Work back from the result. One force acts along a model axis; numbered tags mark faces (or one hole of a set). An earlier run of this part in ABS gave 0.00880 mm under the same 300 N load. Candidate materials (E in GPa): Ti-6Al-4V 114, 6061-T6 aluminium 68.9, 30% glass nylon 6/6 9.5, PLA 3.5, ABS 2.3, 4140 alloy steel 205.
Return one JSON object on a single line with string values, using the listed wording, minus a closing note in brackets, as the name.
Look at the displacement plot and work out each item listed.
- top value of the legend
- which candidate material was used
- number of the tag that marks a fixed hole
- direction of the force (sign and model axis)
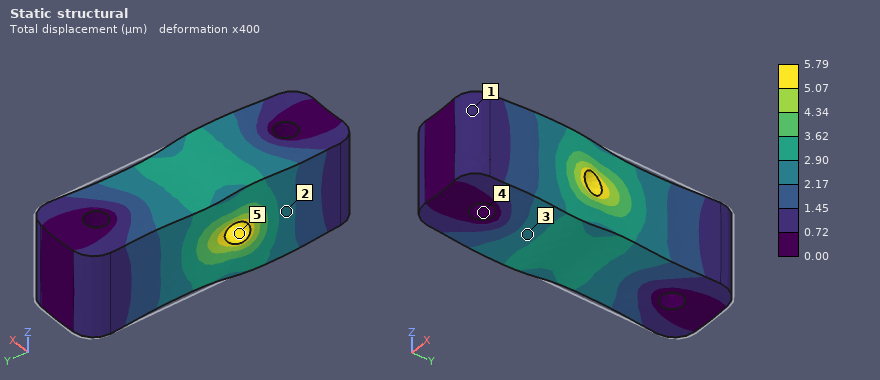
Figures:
{"top value of the legend": "5.79 µm", "which candidate material was used": "PLA", "number of the tag that marks a fixed hole": "4", "direction of the force": "-Y"}
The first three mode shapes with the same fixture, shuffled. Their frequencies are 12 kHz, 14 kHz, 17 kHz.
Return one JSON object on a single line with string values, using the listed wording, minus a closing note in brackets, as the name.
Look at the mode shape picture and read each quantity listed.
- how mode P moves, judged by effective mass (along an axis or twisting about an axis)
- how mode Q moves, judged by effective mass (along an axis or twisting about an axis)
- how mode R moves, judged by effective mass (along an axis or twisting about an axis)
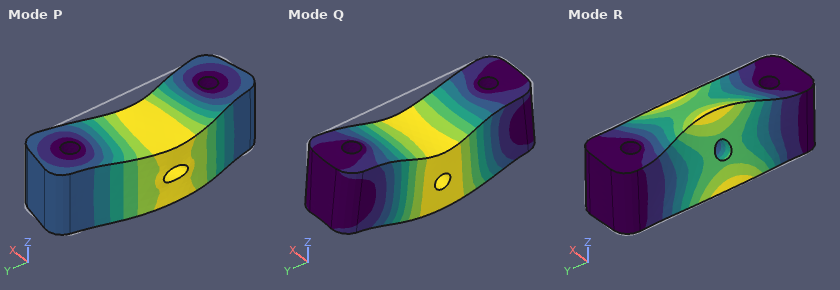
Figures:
{"how mode P moves, judged by effective mass": "along X", "how mode Q moves, judged by effective mass": "along Z", "how mode R moves, judged by effective mass": "twisting about Y"}
